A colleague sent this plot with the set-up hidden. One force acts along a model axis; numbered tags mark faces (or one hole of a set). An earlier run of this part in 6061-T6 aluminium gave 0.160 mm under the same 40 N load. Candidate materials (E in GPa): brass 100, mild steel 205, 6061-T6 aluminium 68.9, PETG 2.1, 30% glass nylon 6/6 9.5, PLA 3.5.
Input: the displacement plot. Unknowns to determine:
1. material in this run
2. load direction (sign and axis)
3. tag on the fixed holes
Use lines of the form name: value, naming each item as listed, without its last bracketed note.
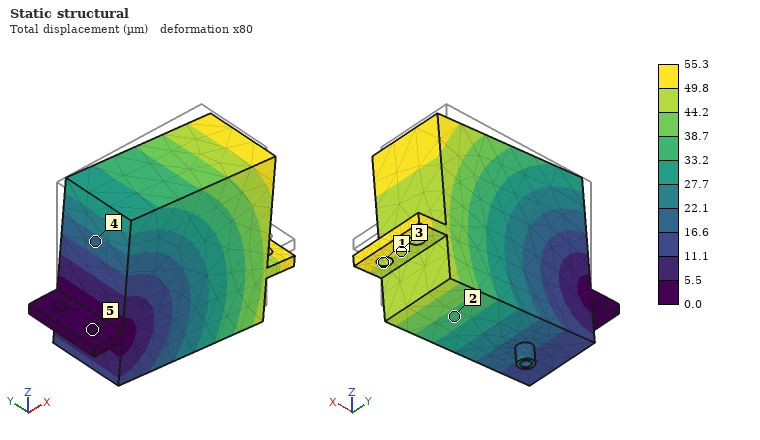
material in this run: mild steel
load direction: -Z
tag on the fixed holes: 5
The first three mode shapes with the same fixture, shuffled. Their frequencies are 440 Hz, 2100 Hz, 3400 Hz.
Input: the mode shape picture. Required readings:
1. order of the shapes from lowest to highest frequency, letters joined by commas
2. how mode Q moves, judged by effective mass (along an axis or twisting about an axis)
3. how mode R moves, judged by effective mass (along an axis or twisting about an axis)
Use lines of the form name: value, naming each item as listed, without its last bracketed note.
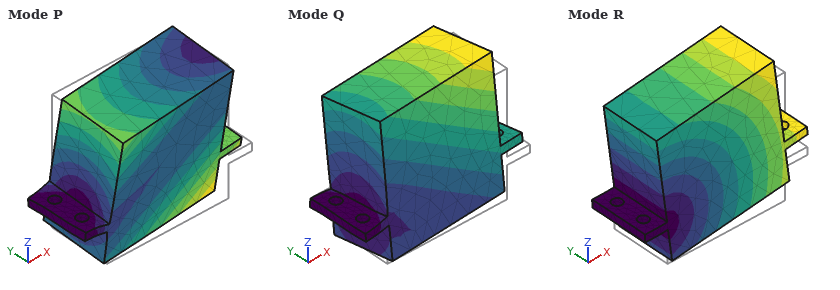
order of the shapes from lowest to highest frequency, letters joined by commas: R, Q, P
how mode Q moves, judged by effective mass: along Y
how mode R moves, judged by effective mass: along Z
